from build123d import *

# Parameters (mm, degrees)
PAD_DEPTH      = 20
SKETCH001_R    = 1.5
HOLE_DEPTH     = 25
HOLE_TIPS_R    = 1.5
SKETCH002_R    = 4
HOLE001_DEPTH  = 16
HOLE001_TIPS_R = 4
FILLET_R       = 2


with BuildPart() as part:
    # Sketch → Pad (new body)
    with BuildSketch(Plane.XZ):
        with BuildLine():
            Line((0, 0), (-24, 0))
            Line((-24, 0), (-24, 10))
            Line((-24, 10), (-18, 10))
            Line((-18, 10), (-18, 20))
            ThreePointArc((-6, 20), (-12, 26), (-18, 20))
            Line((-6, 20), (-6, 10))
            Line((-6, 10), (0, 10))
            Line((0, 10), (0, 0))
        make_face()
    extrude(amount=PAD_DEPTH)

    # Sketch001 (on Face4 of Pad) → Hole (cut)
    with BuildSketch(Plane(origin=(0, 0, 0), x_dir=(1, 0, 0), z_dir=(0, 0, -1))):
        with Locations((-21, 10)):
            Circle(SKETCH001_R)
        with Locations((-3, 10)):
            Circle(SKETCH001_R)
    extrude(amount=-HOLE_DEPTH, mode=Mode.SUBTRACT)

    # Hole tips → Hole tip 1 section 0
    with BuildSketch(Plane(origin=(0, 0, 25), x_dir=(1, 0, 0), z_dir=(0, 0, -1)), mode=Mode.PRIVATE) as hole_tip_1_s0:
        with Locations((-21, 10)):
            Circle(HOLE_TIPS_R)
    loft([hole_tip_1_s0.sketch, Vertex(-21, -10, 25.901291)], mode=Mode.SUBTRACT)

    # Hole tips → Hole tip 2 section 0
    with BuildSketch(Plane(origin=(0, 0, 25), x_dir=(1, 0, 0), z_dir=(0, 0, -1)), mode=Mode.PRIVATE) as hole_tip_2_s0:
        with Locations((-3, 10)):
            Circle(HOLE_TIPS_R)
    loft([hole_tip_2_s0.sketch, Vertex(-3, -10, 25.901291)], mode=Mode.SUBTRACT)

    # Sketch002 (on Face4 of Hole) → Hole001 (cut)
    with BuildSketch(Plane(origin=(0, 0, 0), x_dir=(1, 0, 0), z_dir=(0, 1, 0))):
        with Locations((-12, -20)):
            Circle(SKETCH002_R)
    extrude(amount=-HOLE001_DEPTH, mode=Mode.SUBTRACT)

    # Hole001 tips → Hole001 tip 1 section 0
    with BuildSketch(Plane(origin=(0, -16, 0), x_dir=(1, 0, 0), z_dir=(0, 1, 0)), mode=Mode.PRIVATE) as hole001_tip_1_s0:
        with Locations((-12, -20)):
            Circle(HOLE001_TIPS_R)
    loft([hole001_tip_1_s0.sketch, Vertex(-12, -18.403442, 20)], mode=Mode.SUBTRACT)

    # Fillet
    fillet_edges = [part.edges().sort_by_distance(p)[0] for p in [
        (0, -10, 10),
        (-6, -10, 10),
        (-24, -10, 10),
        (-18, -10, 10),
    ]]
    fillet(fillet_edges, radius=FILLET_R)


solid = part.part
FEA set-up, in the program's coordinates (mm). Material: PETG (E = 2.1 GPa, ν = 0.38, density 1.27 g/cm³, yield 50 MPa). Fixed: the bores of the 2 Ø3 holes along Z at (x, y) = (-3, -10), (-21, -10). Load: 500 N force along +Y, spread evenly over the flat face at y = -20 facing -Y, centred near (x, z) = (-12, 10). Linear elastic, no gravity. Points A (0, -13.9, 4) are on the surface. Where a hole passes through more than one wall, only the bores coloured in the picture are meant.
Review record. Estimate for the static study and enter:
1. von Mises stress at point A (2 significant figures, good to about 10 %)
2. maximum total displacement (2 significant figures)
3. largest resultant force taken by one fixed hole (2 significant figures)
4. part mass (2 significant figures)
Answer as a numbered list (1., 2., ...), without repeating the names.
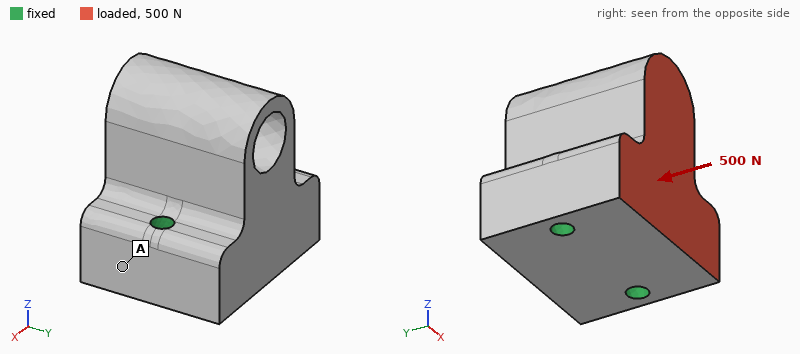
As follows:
1. 1.7 MPa
2. 0.11 mm
3. 250 N
4. 9.3 g
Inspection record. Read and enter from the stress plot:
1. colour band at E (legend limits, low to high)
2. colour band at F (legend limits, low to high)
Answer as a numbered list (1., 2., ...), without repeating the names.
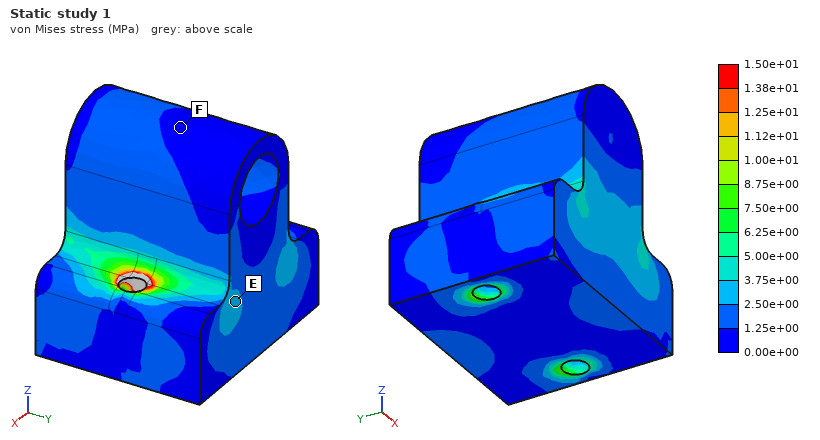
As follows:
1. 2.50e+00 to 3.75e+00 MPa
2. 0.00e+00 to 1.25e+00 MPa
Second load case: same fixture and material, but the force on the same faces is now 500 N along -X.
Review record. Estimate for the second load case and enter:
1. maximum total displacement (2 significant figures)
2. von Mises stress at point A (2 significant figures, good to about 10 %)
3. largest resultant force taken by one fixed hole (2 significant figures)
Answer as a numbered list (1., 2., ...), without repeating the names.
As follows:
1. 0.10 mm
2. 3.0 MPa
3. 380 N
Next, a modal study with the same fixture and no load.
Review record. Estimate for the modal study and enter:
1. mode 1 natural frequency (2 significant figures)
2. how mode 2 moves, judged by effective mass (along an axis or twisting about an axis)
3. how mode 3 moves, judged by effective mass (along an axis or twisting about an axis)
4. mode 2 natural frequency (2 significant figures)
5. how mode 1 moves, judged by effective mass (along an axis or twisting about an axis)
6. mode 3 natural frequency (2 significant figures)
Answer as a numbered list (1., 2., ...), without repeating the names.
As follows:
1. 4600 Hz
2. along X
3. along Z
4. 6100 Hz
5. along Y
6. 9600 Hz
